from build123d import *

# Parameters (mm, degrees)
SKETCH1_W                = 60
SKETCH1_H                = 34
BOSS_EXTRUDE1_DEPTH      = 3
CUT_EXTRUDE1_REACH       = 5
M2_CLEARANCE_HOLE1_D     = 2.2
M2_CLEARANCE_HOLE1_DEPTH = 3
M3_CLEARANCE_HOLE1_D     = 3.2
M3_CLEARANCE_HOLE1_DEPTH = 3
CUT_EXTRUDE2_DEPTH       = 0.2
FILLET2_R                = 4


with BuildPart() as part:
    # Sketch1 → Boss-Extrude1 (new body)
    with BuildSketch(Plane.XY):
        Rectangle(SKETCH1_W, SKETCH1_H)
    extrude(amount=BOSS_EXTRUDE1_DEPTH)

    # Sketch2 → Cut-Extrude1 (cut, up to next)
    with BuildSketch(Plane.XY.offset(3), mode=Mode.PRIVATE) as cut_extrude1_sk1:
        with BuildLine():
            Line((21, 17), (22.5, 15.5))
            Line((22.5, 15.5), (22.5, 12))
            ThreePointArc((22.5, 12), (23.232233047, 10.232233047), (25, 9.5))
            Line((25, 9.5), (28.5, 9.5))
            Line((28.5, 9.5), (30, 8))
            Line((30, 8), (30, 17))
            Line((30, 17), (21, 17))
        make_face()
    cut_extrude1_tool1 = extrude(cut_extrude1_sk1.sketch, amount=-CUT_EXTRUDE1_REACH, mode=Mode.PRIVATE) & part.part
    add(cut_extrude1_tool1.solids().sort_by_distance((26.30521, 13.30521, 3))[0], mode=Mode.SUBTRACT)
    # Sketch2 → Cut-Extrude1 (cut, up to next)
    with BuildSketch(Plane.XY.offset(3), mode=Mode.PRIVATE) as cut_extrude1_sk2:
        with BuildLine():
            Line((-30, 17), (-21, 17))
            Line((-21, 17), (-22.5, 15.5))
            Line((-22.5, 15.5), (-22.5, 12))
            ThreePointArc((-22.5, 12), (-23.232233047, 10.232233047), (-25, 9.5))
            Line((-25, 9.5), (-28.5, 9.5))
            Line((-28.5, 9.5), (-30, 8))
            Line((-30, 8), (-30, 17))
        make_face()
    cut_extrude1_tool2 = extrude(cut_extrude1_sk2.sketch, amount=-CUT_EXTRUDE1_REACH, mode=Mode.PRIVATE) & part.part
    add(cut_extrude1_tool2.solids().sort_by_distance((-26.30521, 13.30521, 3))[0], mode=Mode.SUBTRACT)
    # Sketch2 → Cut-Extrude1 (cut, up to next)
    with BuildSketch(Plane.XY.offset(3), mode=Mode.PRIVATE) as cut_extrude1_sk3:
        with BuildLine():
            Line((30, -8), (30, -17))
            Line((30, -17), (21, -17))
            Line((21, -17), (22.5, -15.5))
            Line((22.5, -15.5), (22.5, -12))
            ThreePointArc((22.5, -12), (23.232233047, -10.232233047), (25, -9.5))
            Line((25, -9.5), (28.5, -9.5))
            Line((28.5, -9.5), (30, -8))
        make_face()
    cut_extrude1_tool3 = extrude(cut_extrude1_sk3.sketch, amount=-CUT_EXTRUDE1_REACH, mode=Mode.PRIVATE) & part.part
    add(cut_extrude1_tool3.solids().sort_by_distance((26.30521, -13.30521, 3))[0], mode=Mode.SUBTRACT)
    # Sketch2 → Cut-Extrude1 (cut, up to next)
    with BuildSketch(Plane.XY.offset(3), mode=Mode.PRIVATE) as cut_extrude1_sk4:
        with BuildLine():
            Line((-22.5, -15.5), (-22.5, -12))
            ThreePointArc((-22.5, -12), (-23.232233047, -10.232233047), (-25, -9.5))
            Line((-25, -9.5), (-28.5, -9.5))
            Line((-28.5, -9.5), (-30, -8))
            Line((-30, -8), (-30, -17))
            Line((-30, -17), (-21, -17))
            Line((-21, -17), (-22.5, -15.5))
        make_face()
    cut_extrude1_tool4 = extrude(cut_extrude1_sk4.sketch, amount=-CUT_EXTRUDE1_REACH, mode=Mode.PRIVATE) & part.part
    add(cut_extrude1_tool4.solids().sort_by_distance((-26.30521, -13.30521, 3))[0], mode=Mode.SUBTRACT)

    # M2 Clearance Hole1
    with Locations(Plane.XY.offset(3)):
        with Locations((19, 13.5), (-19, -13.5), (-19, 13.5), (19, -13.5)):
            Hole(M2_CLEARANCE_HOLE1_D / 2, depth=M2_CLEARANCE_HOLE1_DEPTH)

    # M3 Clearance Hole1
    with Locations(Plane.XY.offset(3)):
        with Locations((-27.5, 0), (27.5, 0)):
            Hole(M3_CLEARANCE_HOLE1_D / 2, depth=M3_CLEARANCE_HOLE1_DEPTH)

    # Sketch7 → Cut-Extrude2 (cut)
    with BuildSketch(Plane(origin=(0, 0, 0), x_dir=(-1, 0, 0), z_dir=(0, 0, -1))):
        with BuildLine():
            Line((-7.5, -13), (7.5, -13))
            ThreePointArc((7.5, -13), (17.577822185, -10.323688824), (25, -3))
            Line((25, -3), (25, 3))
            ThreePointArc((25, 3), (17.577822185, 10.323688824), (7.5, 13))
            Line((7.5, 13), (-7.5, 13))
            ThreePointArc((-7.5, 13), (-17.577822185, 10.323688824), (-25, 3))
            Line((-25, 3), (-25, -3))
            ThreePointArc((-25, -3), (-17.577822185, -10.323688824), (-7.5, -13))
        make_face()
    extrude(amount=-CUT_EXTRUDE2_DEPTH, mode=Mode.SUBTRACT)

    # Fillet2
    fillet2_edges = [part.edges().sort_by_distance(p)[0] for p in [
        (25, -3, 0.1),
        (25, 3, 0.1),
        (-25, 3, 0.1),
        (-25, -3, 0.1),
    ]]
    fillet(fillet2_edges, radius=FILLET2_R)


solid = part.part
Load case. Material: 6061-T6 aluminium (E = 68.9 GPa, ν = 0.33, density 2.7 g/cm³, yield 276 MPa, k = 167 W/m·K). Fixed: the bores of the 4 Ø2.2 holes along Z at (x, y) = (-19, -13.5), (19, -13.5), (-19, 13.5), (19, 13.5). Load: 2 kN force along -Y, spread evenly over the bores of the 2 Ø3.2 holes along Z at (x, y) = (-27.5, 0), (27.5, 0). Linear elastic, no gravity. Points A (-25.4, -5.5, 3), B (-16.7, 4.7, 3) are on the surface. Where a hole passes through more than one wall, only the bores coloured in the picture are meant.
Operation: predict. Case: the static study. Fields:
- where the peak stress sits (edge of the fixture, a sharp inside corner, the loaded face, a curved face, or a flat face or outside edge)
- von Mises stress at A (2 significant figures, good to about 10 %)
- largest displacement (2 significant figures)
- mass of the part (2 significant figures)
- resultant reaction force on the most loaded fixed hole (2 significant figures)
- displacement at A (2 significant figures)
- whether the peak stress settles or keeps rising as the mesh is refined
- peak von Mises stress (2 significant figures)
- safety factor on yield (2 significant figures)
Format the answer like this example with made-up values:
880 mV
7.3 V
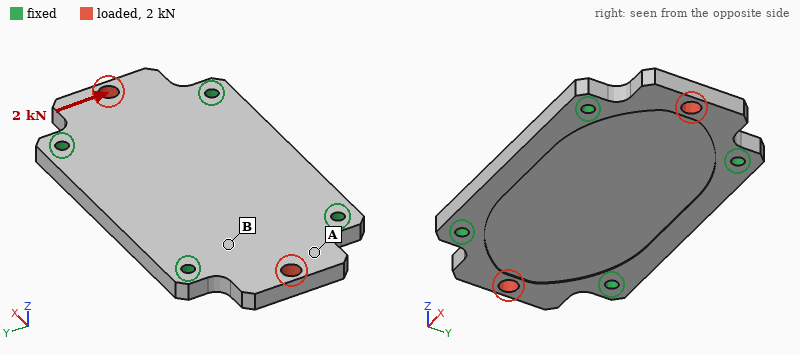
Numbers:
a curved face
30 MPa
11 µm
14 g
560 N
5.8 µm
settles
87 MPa
3.2
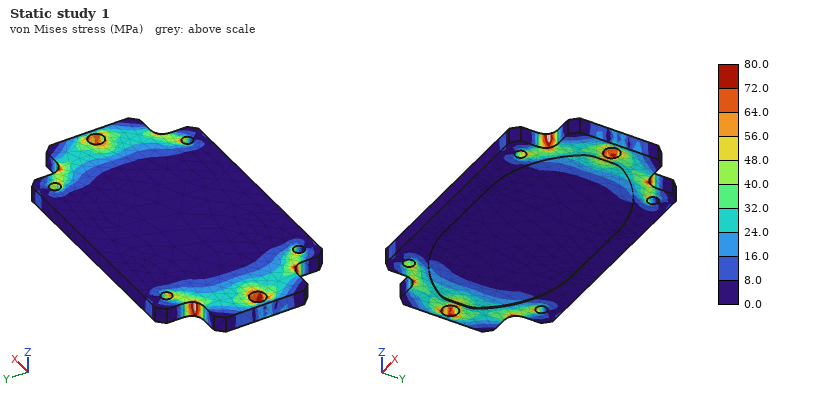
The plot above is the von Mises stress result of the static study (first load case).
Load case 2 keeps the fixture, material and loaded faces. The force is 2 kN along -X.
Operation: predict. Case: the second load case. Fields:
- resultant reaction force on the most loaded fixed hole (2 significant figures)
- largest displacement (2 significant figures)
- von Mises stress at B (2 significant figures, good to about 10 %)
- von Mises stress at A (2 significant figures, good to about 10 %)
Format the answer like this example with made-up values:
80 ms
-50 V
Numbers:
510 N
13 µm
14 MPa
21 MPa
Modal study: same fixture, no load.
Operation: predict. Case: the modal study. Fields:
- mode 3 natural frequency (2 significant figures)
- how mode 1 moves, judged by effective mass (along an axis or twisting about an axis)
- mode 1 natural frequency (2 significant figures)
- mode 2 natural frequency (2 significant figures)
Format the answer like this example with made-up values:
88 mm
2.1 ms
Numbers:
12 kHz
along Z
8300 Hz
12 kHz
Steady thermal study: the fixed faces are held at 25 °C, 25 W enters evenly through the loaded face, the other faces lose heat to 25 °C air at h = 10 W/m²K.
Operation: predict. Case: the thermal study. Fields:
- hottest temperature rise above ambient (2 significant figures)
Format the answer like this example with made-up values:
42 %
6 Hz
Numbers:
26 K
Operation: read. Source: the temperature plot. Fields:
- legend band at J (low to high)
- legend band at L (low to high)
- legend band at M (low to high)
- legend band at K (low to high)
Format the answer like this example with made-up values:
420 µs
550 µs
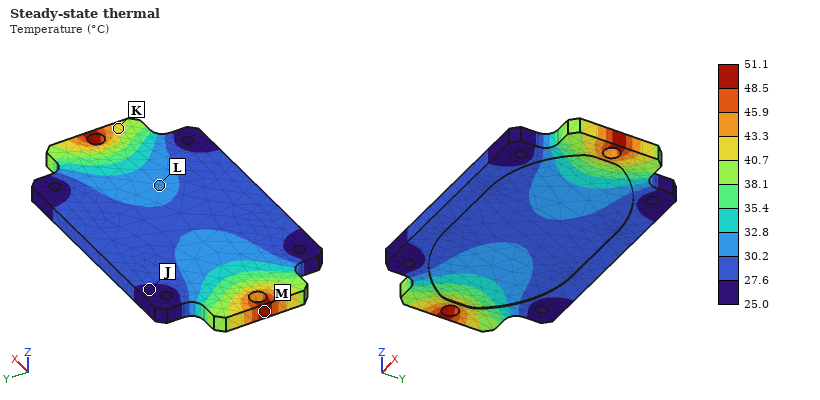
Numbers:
25.0 to 27.6 °C
30.2 to 32.8 °C
48.5 to 51.1 °C
40.7 to 43.3 °C
